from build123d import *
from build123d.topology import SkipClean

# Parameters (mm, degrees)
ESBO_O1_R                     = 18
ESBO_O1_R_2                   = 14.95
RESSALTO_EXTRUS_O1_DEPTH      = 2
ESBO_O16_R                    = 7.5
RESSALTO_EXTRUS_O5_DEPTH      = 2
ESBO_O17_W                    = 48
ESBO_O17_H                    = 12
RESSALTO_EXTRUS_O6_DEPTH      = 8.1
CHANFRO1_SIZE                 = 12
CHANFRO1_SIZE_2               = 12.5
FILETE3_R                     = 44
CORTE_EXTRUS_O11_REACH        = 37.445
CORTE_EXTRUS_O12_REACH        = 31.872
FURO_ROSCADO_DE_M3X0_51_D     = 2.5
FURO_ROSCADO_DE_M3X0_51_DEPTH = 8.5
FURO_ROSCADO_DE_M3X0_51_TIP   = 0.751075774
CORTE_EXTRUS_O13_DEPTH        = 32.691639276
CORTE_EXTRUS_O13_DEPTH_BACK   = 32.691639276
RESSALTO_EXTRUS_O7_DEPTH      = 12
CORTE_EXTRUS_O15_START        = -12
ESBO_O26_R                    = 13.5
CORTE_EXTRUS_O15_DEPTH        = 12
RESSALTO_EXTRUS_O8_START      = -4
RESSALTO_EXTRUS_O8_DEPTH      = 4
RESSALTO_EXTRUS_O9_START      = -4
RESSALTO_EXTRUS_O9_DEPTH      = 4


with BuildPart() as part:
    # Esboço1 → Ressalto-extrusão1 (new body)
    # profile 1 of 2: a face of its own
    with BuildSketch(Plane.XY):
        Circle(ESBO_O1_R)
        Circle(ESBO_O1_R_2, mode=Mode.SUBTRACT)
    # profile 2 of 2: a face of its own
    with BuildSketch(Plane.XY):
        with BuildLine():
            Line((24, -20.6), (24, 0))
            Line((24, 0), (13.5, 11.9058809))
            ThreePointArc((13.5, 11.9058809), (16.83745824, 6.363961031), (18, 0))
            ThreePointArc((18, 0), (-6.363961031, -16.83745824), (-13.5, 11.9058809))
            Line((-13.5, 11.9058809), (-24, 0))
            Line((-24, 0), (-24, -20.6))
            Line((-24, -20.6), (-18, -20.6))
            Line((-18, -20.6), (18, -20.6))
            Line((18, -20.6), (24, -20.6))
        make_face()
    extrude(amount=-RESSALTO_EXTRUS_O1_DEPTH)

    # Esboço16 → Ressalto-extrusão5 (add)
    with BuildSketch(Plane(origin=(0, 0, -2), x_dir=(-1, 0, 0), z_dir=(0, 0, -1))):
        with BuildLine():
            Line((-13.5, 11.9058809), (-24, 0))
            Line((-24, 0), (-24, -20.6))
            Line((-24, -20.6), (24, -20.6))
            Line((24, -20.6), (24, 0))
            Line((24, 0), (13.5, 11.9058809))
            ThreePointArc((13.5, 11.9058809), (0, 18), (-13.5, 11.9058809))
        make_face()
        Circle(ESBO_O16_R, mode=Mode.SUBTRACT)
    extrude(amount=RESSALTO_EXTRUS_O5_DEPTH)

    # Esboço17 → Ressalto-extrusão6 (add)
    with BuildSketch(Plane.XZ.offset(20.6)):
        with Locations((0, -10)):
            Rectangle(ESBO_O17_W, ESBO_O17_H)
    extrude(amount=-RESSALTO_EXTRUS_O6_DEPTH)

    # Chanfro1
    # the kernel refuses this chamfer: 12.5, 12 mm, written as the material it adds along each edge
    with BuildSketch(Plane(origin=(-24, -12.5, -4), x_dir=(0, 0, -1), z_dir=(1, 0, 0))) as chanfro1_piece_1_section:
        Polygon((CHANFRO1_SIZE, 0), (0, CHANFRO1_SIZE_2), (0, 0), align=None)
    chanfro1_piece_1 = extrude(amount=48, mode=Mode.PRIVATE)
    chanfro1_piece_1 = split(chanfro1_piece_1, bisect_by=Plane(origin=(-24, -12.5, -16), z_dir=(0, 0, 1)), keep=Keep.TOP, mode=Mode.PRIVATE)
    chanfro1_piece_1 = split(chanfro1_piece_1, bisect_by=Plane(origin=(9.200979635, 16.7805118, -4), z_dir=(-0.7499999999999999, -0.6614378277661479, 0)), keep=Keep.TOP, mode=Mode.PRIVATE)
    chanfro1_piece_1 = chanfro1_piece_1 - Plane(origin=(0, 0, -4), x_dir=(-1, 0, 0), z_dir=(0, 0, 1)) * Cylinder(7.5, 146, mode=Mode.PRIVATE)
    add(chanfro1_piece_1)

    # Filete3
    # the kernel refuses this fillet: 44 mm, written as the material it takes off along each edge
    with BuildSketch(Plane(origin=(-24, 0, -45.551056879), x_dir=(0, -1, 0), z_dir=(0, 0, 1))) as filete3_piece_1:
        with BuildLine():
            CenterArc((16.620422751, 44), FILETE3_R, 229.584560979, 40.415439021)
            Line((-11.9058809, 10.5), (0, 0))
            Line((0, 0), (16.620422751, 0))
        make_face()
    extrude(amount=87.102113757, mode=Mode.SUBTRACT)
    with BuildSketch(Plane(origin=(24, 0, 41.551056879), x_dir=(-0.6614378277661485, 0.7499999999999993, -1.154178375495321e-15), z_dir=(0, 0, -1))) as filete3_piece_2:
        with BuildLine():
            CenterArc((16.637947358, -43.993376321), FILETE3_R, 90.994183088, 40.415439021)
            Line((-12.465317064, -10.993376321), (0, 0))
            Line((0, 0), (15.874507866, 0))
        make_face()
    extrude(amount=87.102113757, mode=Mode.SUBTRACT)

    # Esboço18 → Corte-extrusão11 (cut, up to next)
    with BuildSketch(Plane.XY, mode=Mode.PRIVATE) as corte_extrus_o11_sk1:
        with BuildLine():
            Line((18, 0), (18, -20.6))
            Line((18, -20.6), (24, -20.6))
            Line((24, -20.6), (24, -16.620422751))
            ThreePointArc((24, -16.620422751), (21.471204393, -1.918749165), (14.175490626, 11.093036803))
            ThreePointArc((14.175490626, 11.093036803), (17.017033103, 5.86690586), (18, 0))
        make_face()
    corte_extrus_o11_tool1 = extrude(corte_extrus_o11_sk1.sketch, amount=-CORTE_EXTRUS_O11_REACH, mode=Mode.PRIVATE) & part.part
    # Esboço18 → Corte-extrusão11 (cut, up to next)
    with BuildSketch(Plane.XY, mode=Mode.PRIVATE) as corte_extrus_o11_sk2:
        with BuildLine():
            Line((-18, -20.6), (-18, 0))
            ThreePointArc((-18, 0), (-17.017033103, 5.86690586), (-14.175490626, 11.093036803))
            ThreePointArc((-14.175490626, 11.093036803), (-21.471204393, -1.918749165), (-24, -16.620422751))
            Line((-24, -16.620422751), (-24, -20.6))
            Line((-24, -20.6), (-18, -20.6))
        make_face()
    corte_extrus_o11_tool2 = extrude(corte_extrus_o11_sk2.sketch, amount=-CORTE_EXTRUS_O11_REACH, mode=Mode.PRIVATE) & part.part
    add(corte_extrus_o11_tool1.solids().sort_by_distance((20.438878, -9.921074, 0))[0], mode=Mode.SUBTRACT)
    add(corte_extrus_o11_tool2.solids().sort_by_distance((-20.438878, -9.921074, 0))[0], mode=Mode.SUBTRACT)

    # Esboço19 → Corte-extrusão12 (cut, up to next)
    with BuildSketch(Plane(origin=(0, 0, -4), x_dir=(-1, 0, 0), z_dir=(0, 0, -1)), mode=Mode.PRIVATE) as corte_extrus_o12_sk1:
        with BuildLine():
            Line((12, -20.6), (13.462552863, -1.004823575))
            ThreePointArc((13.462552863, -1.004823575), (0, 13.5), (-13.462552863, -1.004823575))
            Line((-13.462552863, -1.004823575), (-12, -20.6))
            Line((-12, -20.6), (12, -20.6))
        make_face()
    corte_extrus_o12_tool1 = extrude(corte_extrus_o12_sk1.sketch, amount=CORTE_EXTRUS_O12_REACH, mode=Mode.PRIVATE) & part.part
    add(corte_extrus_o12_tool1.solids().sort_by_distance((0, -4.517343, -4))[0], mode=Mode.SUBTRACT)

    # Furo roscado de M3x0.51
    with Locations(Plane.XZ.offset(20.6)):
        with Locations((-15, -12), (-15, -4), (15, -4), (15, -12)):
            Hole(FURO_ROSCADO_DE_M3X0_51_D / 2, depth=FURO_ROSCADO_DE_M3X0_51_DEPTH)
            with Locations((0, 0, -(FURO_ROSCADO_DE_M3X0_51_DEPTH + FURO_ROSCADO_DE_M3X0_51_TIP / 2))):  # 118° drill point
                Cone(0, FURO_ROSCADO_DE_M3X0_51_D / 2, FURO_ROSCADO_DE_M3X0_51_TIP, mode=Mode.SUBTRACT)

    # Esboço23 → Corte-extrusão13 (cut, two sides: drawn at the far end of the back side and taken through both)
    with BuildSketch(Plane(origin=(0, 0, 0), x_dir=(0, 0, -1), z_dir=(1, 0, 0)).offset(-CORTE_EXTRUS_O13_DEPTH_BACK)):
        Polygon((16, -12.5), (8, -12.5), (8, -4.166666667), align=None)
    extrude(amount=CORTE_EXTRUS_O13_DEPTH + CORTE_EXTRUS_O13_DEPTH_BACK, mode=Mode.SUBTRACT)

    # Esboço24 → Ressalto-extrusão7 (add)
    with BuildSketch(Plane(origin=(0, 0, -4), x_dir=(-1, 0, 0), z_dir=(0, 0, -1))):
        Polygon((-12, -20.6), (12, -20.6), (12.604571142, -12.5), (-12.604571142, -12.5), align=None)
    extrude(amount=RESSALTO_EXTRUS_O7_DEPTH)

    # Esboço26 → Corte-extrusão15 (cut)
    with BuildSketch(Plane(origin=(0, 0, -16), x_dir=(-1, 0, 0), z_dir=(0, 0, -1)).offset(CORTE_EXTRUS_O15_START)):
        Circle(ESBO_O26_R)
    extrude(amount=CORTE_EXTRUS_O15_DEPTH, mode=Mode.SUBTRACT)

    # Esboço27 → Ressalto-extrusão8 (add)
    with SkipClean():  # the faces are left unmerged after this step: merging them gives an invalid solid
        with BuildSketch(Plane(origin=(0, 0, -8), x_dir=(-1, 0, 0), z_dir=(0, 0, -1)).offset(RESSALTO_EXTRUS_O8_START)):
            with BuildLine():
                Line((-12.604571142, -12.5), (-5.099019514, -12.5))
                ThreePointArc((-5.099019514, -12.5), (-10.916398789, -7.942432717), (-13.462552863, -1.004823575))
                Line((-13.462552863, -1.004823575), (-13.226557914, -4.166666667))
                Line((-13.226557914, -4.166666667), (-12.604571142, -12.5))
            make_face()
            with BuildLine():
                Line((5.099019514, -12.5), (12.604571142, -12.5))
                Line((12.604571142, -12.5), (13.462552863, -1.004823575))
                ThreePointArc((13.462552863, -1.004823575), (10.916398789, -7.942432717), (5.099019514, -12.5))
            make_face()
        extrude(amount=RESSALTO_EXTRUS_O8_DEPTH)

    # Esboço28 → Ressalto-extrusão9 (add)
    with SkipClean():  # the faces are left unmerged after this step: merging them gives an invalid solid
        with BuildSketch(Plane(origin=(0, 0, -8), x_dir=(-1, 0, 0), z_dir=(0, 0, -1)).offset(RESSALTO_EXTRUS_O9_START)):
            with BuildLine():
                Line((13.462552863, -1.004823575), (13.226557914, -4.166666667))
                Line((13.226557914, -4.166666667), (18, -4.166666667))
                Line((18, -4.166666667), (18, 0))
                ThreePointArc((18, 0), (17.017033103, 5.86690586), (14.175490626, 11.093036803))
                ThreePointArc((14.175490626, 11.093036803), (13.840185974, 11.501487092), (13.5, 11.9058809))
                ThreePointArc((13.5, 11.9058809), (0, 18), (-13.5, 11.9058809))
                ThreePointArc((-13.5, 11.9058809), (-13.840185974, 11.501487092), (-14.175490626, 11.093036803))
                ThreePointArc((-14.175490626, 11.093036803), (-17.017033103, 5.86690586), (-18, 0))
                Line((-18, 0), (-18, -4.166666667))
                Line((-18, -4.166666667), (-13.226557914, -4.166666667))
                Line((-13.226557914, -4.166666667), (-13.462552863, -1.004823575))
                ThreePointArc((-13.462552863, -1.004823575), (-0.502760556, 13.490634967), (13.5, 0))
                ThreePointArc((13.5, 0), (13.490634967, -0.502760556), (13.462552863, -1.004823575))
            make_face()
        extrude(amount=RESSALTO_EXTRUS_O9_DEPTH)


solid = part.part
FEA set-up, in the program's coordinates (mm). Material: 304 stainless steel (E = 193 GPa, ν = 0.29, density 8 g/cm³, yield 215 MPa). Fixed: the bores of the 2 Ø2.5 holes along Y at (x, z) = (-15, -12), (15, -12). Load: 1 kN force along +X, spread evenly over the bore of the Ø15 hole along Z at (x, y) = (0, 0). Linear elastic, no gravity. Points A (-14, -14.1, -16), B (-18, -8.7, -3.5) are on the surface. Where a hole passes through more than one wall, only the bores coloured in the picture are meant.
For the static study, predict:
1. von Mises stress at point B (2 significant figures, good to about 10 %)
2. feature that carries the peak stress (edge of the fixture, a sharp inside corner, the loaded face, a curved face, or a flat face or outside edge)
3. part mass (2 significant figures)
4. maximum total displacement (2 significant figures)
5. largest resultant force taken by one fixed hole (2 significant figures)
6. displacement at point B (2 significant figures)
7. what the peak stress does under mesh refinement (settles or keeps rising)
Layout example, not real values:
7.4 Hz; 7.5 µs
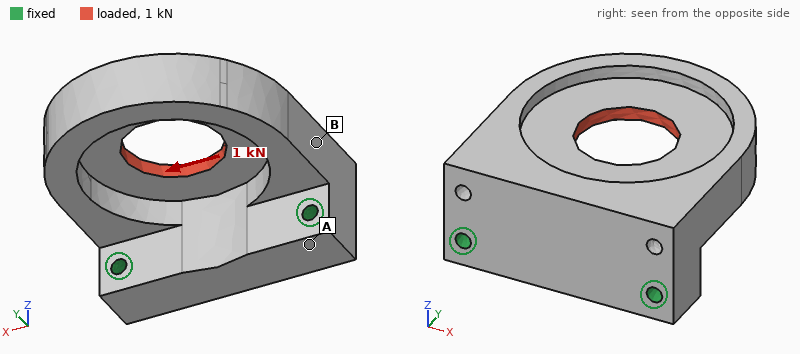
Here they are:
19 MPa; edge of the fixture; 65 g; 10 µm; 760 N; 3.5 µm; keeps rising
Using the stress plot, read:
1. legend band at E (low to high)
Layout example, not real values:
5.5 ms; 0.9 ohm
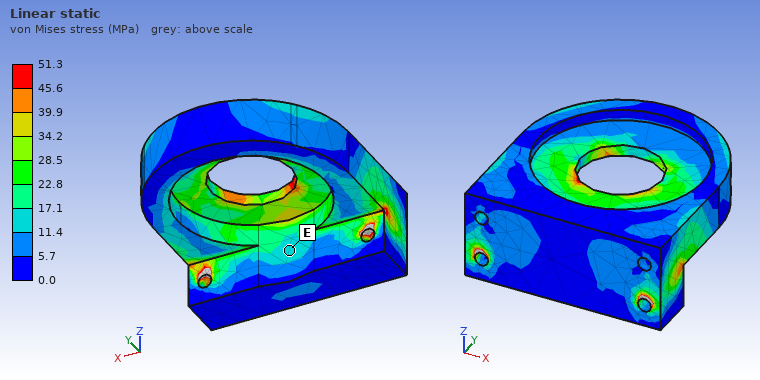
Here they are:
11.4 to 17.1 MPa
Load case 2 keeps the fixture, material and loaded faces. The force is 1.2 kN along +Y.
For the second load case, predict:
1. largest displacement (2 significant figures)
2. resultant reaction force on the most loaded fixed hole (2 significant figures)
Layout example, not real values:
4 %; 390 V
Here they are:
18 µm; 600 N
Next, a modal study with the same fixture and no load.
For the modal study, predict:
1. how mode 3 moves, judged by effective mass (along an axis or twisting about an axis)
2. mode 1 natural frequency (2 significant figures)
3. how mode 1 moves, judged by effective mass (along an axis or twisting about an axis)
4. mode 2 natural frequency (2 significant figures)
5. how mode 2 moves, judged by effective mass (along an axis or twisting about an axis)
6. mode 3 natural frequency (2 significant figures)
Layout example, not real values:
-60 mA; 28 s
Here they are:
along X; 3900 Hz; along Z; 8500 Hz; along X; 12 kHz
